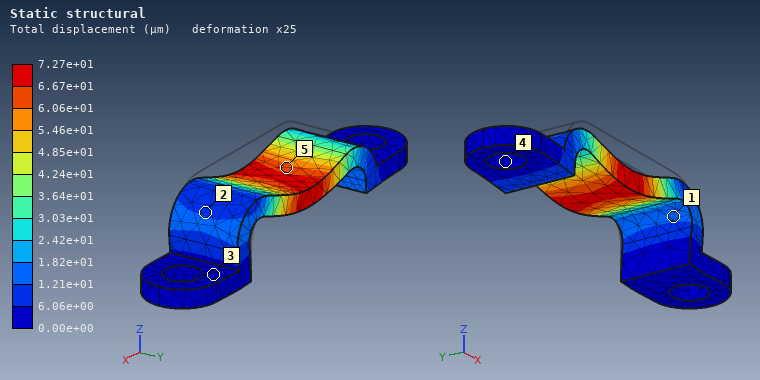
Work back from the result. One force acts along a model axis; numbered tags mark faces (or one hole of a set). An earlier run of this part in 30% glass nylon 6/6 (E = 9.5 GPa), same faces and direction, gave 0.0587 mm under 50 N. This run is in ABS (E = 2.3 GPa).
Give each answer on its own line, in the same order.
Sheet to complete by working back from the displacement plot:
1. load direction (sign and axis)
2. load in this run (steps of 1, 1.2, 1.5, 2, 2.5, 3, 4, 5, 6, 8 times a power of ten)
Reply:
-Z
15 N
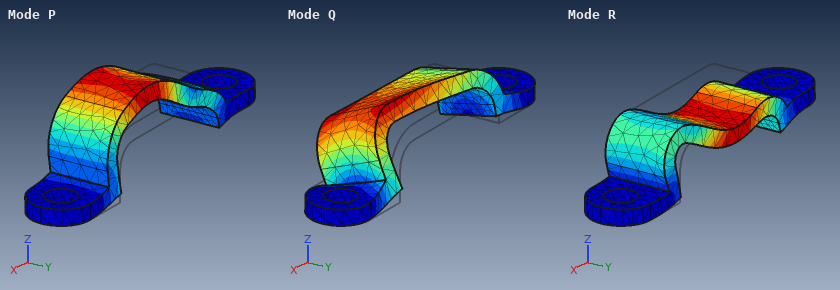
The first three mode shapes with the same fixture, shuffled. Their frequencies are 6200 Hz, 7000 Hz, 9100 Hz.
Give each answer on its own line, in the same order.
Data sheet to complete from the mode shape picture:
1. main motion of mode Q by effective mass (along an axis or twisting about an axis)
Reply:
along Y
